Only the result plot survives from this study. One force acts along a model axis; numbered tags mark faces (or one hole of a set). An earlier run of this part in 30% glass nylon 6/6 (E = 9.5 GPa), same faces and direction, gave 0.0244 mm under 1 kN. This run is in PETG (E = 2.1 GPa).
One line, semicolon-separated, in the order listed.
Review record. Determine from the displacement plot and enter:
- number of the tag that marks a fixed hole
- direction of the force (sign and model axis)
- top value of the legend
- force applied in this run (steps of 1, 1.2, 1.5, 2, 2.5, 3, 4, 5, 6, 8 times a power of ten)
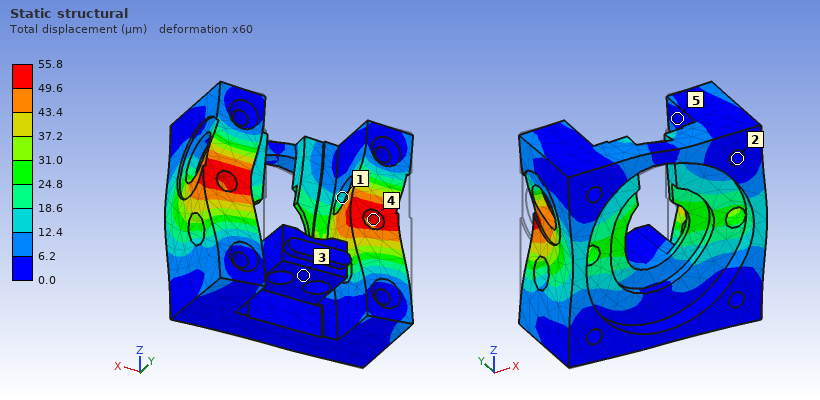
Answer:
2; +X; 55.8 µm; 500 N
